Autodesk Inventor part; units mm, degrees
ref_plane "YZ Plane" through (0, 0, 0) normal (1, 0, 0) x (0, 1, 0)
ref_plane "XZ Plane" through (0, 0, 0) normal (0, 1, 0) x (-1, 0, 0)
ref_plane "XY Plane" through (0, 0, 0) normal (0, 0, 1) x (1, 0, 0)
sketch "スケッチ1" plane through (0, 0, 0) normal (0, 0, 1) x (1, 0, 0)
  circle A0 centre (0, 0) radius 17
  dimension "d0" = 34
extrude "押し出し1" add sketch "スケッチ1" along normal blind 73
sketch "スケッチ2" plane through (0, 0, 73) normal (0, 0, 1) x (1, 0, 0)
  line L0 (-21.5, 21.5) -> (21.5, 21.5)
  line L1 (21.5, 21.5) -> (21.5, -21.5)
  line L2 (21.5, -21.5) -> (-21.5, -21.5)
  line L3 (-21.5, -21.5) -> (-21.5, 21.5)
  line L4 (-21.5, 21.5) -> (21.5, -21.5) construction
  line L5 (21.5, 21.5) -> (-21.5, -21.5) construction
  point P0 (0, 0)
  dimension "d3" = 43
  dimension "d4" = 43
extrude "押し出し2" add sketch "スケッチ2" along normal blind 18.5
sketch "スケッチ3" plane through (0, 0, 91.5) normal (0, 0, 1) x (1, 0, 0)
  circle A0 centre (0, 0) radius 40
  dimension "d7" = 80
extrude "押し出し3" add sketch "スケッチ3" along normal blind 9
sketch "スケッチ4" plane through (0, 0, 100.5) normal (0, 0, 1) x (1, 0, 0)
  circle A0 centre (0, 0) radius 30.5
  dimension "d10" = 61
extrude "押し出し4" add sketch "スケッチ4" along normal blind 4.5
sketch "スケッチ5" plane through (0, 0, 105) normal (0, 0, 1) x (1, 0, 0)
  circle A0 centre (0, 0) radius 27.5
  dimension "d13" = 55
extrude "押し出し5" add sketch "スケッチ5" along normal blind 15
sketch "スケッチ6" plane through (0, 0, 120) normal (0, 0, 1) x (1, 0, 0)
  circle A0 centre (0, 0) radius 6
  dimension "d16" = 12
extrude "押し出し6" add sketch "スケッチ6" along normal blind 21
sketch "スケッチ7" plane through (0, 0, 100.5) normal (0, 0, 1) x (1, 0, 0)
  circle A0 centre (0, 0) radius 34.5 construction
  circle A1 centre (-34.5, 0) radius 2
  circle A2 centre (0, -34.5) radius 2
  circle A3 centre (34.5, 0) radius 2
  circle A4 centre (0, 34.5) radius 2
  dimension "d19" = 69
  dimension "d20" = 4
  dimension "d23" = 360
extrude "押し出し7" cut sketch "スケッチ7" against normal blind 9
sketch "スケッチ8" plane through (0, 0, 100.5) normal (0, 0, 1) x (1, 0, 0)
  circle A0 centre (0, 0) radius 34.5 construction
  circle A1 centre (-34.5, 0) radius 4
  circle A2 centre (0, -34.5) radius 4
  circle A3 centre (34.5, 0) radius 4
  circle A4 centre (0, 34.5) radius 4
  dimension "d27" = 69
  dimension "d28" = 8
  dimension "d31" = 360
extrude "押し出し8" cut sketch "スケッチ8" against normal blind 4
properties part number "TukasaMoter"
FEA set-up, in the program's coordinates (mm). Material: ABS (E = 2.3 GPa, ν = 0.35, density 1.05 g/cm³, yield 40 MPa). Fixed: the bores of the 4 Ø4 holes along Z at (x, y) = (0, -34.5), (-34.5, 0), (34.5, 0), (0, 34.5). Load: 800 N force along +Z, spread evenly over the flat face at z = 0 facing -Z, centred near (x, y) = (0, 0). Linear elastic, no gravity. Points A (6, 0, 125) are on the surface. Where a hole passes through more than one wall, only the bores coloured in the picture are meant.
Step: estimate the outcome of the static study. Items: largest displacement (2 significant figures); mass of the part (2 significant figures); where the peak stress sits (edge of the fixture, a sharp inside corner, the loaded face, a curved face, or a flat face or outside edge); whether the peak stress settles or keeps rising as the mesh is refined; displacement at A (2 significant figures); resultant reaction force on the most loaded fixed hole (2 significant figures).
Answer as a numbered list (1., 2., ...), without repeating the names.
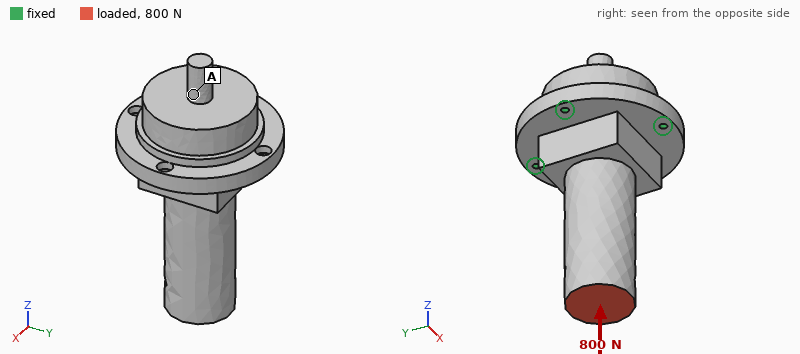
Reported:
1. 63 µm
2. 210 g
3. edge of the fixture
4. keeps rising
5. 29 µm
6. 210 N
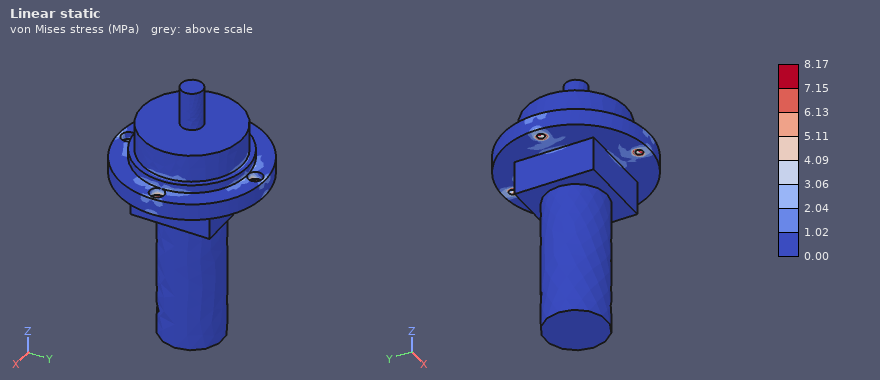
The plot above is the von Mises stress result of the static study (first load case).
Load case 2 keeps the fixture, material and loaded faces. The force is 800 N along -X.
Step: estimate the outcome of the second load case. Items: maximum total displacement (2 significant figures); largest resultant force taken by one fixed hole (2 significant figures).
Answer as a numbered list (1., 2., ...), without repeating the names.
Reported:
1. 1.7 mm
2. 1.1 kN
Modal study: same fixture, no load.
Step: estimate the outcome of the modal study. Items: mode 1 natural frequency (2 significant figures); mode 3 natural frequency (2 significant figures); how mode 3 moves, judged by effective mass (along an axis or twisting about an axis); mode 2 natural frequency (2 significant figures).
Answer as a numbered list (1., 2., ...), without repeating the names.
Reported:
1. 700 Hz
2. 1800 Hz
3. along Z
4. 700 Hz
